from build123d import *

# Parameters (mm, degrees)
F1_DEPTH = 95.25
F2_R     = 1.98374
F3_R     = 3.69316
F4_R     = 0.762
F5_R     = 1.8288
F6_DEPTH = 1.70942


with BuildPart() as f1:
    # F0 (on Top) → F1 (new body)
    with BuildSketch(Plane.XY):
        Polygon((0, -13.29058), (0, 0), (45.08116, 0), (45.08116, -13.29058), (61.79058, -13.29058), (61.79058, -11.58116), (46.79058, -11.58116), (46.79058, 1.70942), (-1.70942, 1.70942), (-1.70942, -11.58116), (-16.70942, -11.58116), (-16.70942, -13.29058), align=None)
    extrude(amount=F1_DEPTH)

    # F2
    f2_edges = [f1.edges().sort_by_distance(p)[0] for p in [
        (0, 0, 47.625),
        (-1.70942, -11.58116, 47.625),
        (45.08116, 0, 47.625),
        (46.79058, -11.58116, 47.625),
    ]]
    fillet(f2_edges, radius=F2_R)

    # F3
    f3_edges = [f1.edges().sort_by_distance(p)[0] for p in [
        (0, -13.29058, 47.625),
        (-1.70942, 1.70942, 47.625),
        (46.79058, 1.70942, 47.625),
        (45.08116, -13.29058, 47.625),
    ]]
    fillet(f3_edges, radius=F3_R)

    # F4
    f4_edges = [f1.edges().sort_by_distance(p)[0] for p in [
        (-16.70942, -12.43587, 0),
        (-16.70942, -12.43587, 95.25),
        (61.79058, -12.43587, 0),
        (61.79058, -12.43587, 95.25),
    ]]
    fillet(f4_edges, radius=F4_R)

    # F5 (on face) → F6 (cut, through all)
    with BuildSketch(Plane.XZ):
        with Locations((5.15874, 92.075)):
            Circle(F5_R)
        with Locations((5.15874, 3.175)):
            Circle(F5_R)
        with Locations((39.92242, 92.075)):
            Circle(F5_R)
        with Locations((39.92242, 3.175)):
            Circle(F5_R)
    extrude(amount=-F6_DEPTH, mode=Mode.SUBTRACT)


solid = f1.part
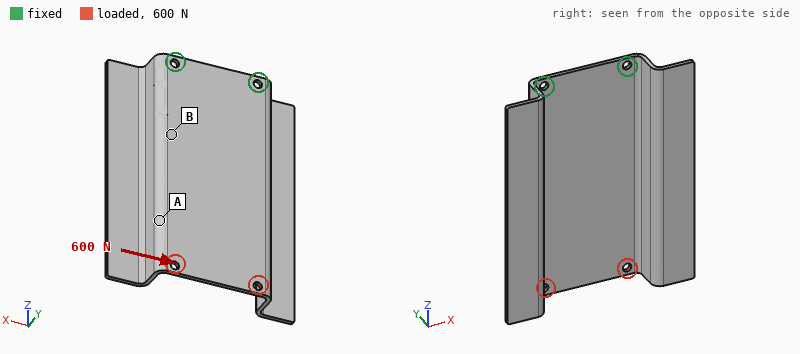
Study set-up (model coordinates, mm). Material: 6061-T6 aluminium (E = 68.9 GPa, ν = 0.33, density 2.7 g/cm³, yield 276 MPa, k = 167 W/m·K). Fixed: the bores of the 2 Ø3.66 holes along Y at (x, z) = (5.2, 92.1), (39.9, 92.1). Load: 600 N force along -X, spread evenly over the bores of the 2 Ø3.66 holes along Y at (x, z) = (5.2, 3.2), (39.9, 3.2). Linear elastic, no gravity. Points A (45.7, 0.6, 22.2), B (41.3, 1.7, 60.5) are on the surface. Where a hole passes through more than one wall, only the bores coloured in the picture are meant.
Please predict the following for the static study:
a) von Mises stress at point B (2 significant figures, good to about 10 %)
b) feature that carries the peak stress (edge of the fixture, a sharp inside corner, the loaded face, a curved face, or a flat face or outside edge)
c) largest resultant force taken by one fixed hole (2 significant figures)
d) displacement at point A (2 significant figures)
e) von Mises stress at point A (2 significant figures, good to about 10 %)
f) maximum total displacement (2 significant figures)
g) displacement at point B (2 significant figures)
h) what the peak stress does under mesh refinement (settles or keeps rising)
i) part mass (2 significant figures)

35 MPa
edge of the fixture
1.5 kN
0.12 mm
14 MPa
0.21 mm
0.046 mm
keeps rising
44 g
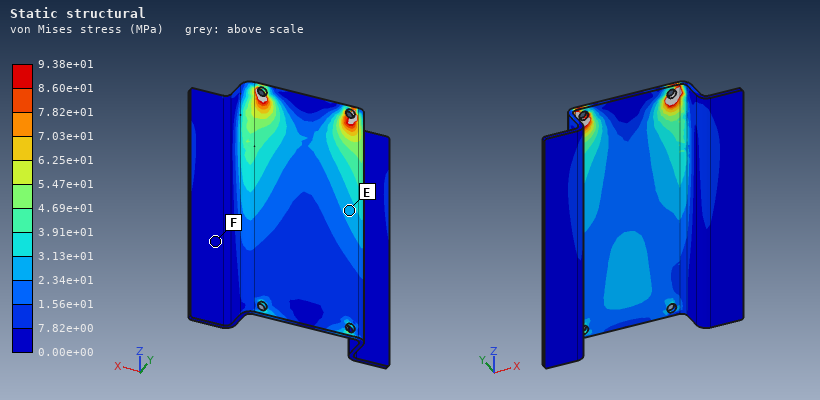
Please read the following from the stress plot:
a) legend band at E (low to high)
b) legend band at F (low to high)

2.34e+01 to 3.13e+01 MPa
0.00e+00 to 7.82e+00 MPa
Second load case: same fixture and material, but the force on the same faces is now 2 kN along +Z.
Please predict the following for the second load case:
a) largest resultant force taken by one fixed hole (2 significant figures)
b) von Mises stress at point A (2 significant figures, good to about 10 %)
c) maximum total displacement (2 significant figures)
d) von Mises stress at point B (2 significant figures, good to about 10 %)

1.0 kN
28 MPa
0.15 mm
25 MPa
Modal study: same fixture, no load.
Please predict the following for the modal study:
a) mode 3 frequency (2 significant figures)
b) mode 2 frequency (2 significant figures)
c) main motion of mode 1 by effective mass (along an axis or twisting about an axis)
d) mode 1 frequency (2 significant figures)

1100 Hz
400 Hz
along Y
280 Hz
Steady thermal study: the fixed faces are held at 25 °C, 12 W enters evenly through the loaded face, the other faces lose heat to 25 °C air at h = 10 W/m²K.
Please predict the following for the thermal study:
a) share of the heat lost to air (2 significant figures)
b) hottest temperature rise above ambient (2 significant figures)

31 %
45 K
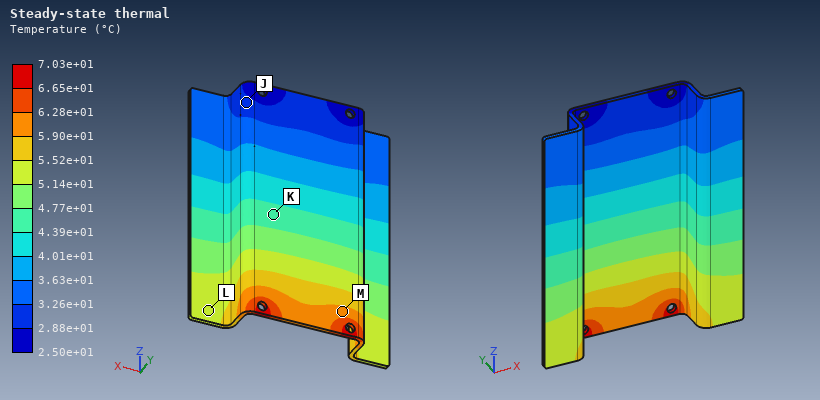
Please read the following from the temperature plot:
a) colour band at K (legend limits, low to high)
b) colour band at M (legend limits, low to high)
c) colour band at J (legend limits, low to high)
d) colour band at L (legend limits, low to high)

4.39e+01 to 4.77e+01 °C
5.90e+01 to 6.28e+01 °C
2.88e+01 to 3.26e+01 °C
5.14e+01 to 5.52e+01 °C
